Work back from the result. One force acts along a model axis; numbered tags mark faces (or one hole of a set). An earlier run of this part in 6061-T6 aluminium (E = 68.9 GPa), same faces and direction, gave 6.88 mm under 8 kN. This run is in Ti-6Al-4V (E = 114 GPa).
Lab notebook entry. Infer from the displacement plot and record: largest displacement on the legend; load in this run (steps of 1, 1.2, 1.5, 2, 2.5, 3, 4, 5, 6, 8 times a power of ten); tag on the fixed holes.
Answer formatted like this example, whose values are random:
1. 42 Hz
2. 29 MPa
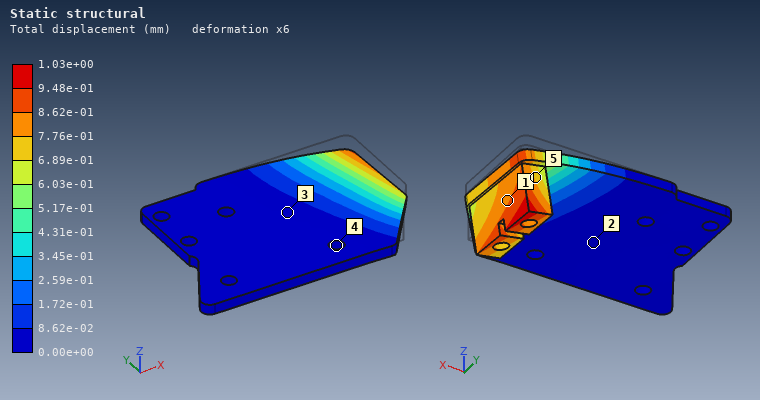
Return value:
1. 1.03e+00 mm
2. 2 kN
3. 4
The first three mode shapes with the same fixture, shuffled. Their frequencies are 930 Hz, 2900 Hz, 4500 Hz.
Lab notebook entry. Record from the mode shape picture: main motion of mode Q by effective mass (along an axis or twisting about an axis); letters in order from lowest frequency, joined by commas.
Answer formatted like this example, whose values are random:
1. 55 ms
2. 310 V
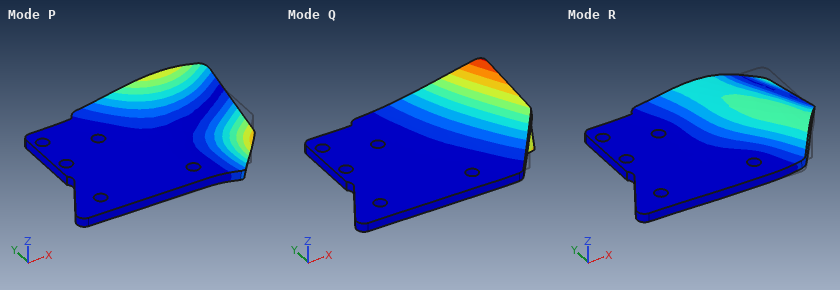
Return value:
1. along Z
2. Q, P, R
